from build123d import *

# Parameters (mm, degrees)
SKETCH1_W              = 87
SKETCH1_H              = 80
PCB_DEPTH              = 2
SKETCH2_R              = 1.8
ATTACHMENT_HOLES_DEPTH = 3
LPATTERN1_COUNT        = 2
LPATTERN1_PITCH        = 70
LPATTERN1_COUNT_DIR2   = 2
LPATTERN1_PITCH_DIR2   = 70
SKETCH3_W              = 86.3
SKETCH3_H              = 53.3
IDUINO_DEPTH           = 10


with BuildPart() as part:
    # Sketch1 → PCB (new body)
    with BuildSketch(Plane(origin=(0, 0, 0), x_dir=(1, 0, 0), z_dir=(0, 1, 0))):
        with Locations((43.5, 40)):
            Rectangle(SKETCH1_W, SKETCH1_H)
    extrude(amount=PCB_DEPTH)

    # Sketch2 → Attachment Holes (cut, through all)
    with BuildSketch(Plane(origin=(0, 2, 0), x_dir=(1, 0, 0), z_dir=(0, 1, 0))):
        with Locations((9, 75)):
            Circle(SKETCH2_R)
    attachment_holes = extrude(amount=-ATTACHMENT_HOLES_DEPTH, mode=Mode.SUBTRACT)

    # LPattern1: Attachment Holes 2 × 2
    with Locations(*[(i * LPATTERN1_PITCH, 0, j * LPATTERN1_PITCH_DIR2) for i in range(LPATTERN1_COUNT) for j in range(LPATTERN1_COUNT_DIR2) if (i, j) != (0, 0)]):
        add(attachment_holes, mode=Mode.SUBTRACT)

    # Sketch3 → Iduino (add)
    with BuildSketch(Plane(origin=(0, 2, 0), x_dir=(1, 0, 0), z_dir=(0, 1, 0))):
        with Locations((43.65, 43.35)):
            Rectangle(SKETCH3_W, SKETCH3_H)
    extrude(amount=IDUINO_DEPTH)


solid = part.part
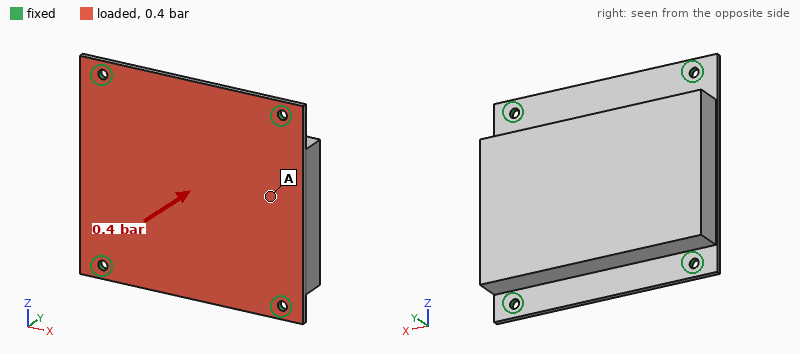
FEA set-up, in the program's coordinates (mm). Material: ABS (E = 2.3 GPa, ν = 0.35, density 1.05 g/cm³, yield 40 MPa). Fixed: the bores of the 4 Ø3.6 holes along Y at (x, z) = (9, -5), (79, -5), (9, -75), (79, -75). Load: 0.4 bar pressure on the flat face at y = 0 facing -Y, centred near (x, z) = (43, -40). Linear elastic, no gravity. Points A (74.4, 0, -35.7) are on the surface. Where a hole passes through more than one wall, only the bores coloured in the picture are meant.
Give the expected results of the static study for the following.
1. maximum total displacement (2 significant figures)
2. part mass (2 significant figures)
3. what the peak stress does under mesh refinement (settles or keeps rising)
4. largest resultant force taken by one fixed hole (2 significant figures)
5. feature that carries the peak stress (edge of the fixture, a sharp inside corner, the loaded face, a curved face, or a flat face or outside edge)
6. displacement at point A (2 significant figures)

0.57 mm
63 g
keeps rising
85 N
edge of the fixture
0.23 mm
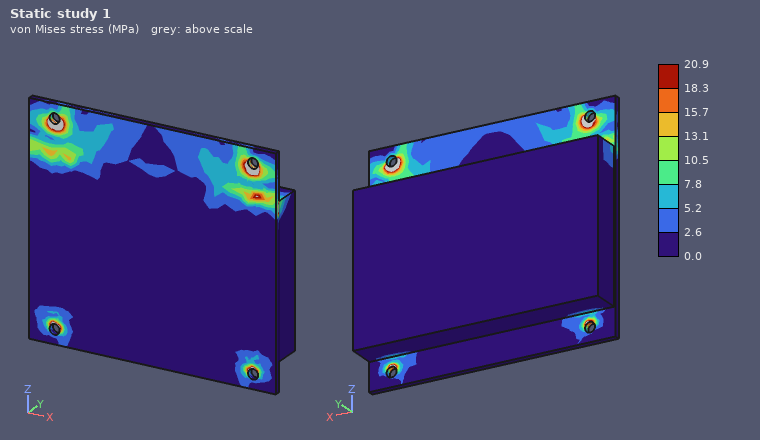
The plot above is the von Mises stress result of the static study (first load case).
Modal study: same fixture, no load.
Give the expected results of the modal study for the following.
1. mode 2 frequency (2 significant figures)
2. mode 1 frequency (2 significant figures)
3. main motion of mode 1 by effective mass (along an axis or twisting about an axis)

1100 Hz
660 Hz
along Y
